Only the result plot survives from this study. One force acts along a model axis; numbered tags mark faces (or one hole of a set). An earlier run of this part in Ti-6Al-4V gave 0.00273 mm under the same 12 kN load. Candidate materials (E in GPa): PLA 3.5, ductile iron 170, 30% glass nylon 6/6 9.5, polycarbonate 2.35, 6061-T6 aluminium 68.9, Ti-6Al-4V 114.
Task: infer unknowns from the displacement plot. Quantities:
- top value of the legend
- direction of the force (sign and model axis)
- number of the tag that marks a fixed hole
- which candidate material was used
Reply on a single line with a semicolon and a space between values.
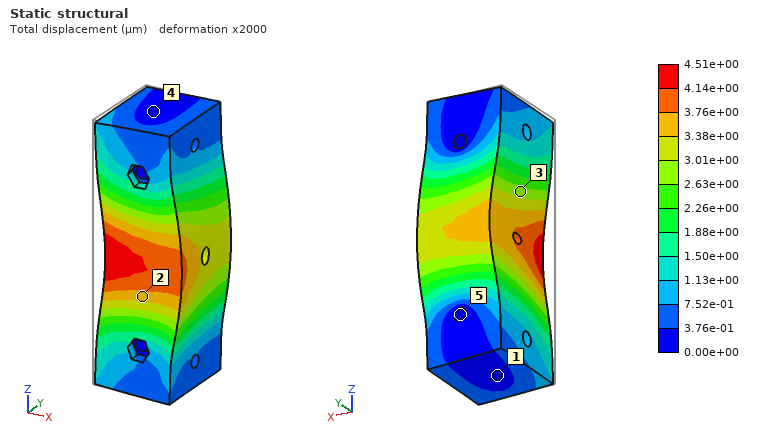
4.51e+00 µm; +X; 5; 6061-T6 aluminium
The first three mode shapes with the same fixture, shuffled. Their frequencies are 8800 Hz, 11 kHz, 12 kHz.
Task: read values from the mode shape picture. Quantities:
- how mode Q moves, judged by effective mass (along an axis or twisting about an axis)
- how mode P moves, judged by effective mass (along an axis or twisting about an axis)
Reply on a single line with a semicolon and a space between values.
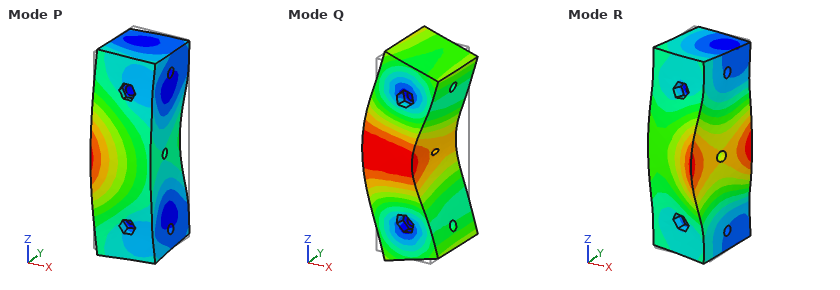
along X; along Y
